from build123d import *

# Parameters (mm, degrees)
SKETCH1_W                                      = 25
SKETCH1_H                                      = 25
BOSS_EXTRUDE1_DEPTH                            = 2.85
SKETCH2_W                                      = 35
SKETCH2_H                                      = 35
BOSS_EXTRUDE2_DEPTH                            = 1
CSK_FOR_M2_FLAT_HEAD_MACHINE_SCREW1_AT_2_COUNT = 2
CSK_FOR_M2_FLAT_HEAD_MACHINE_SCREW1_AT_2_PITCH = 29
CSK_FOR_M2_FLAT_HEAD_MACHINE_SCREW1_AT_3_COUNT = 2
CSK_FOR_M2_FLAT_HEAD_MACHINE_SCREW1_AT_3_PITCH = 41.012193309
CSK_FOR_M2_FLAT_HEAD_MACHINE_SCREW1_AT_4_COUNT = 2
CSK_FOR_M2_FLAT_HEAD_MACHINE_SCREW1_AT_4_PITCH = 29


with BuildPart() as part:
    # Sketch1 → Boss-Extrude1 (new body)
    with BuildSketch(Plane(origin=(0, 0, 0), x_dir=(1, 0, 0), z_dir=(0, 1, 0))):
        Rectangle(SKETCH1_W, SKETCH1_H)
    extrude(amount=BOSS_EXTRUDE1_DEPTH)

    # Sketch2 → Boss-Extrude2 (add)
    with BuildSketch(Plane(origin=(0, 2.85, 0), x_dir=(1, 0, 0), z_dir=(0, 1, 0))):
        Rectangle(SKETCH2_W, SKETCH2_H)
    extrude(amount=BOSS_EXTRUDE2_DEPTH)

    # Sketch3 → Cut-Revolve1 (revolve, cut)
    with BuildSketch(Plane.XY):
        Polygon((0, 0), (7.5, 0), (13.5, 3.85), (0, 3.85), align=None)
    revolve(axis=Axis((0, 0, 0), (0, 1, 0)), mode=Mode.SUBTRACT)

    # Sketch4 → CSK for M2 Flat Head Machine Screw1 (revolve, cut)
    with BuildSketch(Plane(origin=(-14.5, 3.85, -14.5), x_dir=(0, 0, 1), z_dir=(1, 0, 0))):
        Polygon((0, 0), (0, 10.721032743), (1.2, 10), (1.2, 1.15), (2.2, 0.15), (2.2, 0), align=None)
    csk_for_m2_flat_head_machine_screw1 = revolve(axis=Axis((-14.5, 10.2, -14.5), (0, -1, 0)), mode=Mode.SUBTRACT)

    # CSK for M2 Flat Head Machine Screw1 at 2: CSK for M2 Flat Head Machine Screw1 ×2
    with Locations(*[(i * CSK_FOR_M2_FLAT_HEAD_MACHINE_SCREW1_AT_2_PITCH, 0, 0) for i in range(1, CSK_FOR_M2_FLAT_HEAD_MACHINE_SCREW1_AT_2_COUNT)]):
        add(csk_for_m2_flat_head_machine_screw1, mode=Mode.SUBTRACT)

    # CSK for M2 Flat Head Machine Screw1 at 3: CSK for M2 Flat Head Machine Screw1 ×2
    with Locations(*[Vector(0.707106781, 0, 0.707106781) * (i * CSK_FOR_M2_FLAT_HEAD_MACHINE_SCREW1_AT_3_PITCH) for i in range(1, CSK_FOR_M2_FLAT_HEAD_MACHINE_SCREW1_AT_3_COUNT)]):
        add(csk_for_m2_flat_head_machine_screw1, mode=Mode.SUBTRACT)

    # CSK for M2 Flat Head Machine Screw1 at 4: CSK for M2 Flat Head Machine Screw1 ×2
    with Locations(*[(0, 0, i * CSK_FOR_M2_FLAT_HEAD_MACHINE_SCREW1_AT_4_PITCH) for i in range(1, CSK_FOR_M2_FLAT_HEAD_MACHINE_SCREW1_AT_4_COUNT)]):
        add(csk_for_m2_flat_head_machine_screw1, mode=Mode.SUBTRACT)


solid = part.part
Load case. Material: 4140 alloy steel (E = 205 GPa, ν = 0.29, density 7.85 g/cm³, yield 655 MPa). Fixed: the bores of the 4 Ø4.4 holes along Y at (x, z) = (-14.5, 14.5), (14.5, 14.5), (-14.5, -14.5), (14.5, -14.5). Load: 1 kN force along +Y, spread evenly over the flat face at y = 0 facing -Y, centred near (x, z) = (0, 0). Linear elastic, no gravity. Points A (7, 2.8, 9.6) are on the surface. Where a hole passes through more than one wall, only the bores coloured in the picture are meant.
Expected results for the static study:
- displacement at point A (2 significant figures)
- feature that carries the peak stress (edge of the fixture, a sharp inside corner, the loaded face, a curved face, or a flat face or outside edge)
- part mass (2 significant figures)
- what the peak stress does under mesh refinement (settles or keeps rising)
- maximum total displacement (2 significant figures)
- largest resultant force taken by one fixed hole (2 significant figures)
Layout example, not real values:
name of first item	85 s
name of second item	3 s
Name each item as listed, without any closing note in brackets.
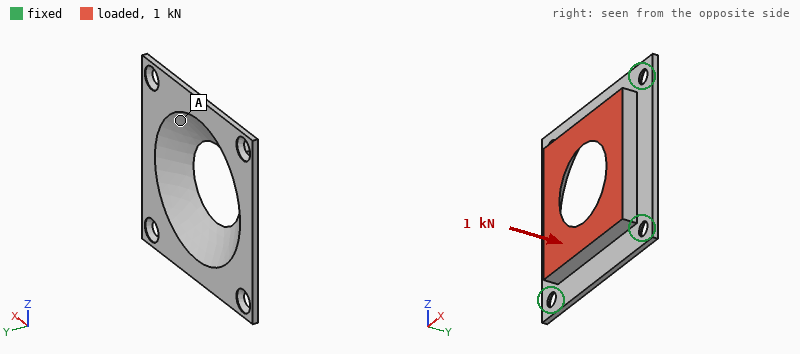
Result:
displacement at point A	13 µm
feature that carries the peak stress	edge of the fixture
part mass	13 g
what the peak stress does under mesh refinement	keeps rising
maximum total displacement	20 µm
largest resultant force taken by one fixed hole	600 N
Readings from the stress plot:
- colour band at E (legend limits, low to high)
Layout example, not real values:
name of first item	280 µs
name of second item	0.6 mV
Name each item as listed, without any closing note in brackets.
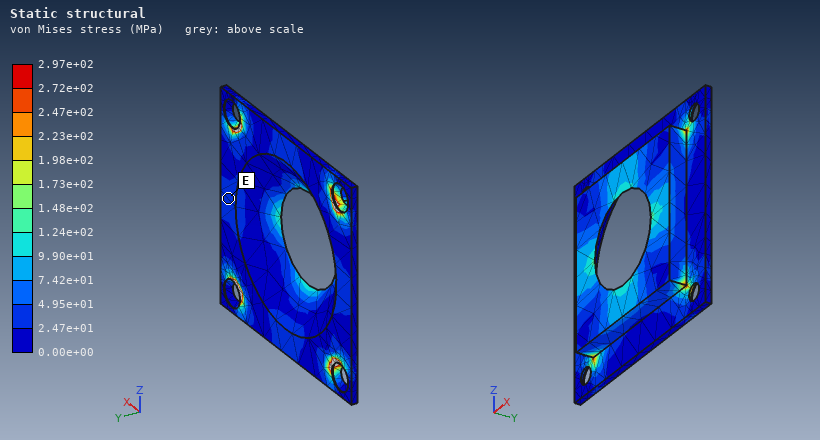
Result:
colour band at E	2.47e+01 to 4.95e+01 MPa
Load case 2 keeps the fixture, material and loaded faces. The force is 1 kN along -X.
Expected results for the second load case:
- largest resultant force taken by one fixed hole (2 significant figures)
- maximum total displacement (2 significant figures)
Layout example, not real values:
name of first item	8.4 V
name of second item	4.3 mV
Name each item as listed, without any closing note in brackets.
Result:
largest resultant force taken by one fixed hole	270 N
maximum total displacement	5.0 µm
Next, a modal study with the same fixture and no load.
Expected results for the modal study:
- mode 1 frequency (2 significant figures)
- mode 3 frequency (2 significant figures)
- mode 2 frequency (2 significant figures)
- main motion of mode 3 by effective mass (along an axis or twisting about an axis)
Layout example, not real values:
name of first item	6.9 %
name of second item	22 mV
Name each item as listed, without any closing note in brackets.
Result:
mode 1 frequency	14 kHz
mode 3 frequency	15 kHz
mode 2 frequency	14 kHz
main motion of mode 3 by effective mass	twisting about Z
